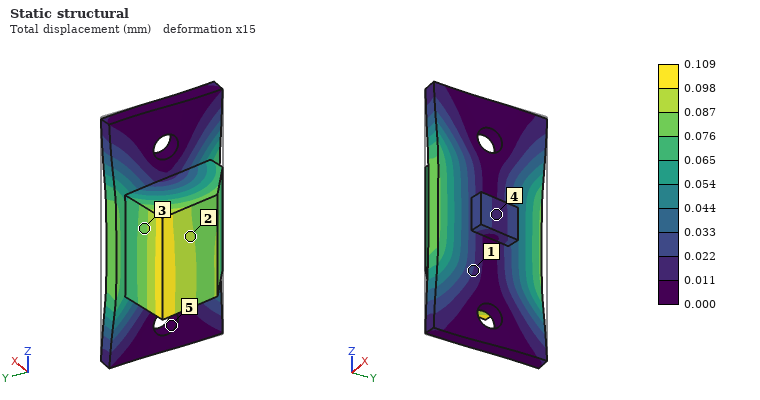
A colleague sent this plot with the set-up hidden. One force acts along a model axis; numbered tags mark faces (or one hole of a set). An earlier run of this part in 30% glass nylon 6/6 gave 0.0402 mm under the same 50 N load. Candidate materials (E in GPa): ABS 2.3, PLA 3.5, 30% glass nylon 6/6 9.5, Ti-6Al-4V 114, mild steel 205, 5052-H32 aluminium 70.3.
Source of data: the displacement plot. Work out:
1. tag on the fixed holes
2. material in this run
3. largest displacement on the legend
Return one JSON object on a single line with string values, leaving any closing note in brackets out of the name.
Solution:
{"tag on the fixed holes": "5", "material in this run": "PLA", "largest displacement on the legend": "0.109 mm"}
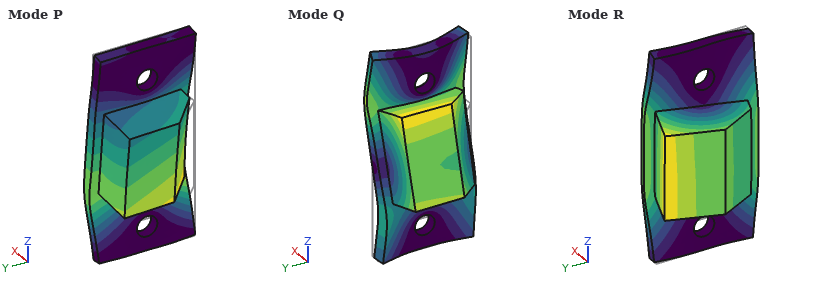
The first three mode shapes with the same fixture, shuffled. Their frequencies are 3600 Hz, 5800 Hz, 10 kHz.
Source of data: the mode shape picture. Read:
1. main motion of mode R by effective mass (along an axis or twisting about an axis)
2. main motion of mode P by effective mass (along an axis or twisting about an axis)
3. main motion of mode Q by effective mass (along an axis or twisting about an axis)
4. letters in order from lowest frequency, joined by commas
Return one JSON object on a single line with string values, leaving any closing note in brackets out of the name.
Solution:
{"main motion of mode R by effective mass": "along Y", "main motion of mode P by effective mass": "along X", "main motion of mode Q by effective mass": "along Z", "letters in order from lowest frequency, joined by commas": "R, P, Q"}
